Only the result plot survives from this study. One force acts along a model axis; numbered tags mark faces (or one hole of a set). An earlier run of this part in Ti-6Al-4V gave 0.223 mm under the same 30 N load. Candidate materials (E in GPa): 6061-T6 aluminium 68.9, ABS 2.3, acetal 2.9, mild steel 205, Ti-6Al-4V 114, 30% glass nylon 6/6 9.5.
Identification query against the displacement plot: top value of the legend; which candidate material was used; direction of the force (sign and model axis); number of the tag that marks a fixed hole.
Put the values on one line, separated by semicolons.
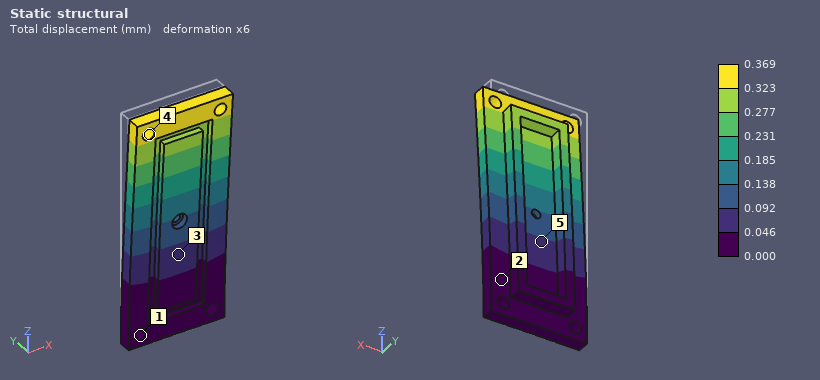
0.369 mm; 6061-T6 aluminium; -Y; 1
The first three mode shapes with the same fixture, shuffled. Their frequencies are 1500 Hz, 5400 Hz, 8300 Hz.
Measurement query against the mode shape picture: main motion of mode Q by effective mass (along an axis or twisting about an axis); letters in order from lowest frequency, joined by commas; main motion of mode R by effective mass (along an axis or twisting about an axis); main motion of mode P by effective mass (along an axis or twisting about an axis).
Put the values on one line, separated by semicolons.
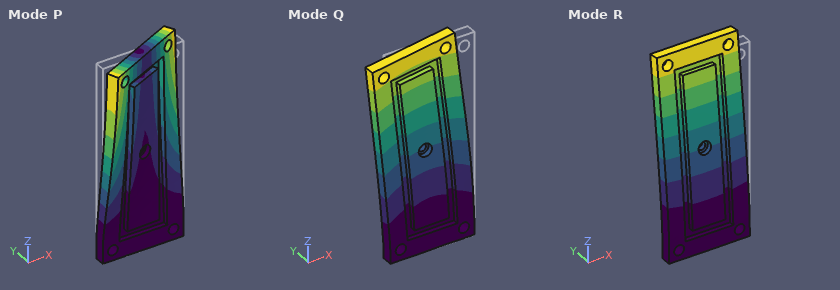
along X; R, P, Q; along Y; twisting about Z
